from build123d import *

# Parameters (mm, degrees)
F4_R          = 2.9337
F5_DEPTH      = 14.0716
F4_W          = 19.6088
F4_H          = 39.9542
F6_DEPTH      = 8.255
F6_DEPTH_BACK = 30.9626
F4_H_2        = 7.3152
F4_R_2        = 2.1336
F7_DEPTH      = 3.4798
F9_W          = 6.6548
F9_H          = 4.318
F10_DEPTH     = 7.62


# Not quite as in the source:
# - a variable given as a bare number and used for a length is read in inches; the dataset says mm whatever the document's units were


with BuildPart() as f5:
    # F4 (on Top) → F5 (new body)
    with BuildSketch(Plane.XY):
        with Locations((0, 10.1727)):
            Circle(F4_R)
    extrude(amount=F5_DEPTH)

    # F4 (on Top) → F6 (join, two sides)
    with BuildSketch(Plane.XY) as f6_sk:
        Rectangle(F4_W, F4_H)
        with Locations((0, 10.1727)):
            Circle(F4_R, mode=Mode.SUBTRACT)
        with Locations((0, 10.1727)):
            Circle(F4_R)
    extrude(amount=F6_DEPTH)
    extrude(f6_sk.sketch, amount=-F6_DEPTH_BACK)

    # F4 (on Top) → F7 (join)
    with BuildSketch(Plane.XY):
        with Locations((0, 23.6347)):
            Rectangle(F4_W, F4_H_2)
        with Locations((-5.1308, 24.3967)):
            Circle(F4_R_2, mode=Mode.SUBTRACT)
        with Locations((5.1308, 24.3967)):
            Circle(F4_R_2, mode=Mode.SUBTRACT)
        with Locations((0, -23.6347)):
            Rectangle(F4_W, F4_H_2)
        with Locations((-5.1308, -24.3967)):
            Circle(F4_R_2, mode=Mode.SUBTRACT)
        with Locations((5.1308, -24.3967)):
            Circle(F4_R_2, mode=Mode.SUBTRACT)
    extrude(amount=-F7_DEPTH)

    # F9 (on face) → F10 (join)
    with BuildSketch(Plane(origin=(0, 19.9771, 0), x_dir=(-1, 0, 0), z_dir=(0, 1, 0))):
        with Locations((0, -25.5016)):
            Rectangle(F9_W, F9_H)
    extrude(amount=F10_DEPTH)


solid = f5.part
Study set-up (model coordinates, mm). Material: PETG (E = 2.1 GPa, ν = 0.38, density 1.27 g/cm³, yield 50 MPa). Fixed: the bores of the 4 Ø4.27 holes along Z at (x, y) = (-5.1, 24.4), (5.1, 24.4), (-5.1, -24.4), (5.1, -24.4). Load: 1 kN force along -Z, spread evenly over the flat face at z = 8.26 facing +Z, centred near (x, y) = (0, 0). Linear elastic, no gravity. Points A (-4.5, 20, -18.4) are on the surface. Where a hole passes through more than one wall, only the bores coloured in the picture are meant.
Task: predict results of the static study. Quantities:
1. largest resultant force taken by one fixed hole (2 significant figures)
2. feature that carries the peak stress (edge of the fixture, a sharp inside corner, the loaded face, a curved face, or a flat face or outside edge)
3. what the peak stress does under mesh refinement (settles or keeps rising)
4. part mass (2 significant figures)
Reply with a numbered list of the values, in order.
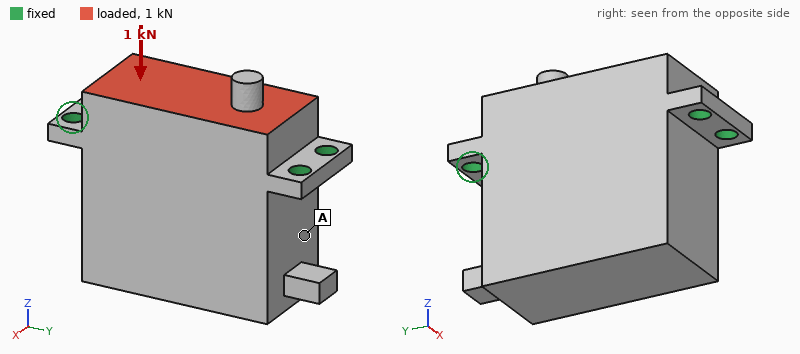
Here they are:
1. 250 N
2. edge of the fixture
3. keeps rising
4. 41 g
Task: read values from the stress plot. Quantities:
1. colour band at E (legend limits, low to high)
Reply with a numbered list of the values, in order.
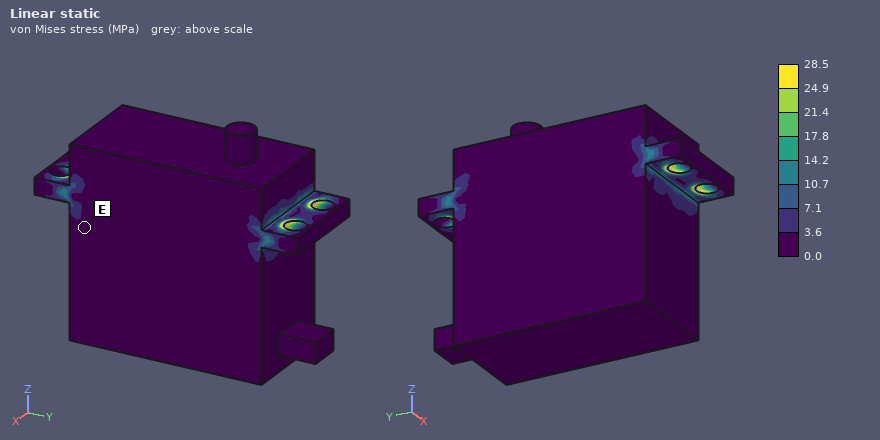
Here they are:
1. 0.0 to 3.6 MPa
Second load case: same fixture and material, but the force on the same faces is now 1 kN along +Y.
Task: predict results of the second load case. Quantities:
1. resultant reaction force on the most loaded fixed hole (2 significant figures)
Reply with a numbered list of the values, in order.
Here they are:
1. 280 N
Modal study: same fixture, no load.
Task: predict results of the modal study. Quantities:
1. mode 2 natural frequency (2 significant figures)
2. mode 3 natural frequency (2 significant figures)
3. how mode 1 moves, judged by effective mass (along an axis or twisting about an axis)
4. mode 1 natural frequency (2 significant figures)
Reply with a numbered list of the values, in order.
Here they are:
1. 2800 Hz
2. 2900 Hz
3. along X
4. 1000 Hz
